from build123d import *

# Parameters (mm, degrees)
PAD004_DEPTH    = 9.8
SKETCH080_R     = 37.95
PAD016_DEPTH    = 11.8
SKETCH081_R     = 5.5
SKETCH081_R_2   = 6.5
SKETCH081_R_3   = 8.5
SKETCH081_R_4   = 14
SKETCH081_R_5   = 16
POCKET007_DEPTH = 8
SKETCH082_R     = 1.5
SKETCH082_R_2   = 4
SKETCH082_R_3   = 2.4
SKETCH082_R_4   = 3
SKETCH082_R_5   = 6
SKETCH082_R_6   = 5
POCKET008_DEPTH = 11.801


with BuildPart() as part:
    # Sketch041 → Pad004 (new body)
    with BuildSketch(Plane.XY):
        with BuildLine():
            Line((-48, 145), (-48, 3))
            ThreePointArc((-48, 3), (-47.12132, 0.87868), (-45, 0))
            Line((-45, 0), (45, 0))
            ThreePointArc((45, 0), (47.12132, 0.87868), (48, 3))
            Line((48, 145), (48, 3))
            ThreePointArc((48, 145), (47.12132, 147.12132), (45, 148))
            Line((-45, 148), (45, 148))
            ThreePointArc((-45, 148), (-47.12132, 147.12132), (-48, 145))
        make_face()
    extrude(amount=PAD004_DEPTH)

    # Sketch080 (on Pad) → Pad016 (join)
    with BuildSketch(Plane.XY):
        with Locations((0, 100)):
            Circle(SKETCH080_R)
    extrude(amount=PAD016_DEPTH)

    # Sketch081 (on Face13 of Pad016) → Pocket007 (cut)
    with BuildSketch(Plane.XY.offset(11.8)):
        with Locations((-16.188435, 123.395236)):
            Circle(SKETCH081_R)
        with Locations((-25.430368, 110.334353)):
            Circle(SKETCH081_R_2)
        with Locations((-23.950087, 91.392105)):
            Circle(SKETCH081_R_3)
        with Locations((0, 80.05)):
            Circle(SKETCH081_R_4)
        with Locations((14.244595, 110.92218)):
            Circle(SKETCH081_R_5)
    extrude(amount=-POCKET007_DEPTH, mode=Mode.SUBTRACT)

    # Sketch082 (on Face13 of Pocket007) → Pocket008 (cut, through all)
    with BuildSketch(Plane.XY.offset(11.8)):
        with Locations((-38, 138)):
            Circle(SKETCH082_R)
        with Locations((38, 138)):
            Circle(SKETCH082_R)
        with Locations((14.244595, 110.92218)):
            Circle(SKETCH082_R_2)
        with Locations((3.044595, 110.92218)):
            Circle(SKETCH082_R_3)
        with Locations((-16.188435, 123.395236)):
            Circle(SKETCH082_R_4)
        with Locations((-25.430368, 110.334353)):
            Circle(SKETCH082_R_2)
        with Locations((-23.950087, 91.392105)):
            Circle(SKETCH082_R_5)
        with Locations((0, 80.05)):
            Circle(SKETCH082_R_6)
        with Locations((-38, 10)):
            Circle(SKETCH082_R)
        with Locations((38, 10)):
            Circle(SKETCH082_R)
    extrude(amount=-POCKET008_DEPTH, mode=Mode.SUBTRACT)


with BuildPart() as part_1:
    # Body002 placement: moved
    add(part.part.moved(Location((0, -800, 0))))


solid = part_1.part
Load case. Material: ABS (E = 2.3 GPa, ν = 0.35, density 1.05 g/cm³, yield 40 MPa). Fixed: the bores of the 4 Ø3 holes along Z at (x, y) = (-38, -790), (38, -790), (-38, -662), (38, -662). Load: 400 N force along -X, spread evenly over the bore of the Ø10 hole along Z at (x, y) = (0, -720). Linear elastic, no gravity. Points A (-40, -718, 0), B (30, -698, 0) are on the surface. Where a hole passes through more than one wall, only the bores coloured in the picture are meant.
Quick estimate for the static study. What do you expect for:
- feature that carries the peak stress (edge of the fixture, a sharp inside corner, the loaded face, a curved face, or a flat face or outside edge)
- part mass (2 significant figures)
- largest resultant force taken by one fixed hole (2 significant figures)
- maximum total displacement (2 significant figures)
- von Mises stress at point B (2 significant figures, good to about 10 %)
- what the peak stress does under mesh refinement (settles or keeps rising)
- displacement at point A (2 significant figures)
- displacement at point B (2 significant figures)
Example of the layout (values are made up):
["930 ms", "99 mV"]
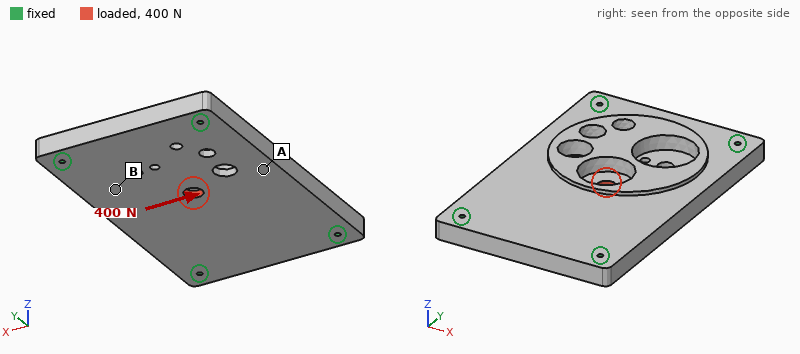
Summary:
["a sharp inside corner", "140 g", "140 N", "47 µm", "0.72 MPa", "keeps rising", "34 µm", "25 µm"]
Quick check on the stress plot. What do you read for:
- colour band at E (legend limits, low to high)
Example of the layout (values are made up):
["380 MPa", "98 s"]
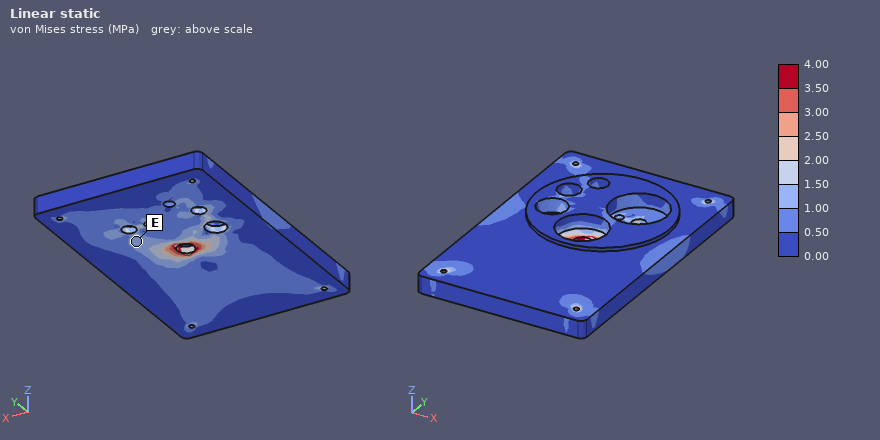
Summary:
["1.00 to 1.50 MPa"]
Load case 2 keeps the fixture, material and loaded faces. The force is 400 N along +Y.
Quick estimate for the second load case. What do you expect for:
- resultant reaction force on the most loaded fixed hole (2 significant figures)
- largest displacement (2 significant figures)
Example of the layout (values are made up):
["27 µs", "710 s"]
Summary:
["110 N", "31 µm"]
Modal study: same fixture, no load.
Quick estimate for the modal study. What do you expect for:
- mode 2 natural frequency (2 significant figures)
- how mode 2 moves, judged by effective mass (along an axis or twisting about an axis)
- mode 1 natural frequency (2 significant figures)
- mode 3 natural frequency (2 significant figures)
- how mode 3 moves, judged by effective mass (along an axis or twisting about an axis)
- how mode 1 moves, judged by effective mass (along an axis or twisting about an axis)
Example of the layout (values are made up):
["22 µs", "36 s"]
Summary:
["1000 Hz", "twisting about Y", "680 Hz", "1700 Hz", "twisting about X", "along Z"]
